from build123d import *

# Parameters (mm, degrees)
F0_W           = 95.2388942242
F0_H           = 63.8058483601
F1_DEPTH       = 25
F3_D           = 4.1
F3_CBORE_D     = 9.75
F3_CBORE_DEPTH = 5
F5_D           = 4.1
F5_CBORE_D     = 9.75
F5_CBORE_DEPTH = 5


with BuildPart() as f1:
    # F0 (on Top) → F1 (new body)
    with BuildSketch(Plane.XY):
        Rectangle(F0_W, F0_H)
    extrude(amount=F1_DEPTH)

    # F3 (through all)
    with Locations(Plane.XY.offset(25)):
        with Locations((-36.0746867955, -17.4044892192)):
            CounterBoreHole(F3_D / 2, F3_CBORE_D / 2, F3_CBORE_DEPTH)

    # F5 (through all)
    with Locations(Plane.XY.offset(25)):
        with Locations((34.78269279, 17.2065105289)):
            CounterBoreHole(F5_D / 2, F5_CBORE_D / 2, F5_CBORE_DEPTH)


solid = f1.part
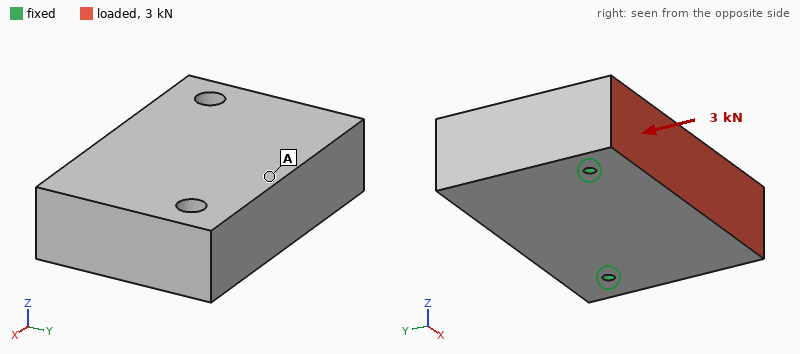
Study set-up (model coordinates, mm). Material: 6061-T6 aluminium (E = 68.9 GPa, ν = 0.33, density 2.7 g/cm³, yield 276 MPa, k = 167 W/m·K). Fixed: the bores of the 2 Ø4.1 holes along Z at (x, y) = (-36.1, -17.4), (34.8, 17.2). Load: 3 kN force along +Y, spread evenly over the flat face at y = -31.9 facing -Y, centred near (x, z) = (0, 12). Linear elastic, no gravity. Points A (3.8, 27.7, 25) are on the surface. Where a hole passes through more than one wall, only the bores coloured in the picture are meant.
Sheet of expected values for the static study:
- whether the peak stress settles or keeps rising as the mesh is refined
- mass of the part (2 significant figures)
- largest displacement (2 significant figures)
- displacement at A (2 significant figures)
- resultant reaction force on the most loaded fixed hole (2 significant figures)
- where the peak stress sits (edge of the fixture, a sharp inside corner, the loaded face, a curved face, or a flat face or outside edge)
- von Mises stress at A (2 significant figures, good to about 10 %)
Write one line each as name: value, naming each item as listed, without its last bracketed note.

whether the peak stress settles or keeps rising as the mesh is refined: keeps rising
mass of the part: 410 g
largest displacement: 2.2 µm
displacement at A: 1.6 µm
resultant reaction force on the most loaded fixed hole: 1.5 kN
where the peak stress sits: edge of the fixture
von Mises stress at A: 0.99 MPa
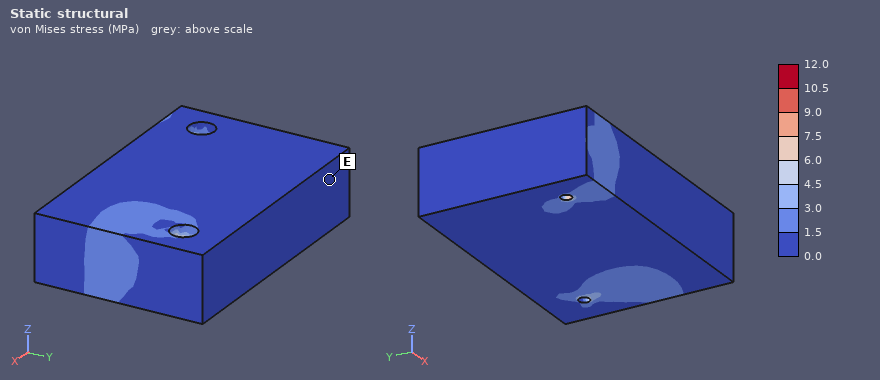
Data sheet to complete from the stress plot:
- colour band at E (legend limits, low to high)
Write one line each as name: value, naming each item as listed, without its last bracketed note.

colour band at E: 0.0 to 1.5 MPa
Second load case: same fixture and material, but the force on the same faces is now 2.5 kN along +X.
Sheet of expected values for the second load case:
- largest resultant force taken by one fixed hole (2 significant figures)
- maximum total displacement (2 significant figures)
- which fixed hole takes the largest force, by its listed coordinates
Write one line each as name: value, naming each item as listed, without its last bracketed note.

largest resultant force taken by one fixed hole: 2.0 kN
maximum total displacement: 3.7 µm
which fixed hole takes the largest force, by its listed coordinates: (-36.1, -17.4)
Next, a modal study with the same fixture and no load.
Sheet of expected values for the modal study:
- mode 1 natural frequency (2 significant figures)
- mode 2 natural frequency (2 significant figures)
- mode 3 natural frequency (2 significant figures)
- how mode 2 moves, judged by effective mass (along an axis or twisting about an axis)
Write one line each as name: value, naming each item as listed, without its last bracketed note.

mode 1 natural frequency: 4900 Hz
mode 2 natural frequency: 7100 Hz
mode 3 natural frequency: 12 kHz
how mode 2 moves, judged by effective mass: along Z
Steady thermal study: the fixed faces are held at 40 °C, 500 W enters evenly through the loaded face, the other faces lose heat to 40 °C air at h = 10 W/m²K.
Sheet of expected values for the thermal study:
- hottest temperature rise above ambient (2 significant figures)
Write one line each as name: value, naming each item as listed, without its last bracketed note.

hottest temperature rise above ambient: 71 K
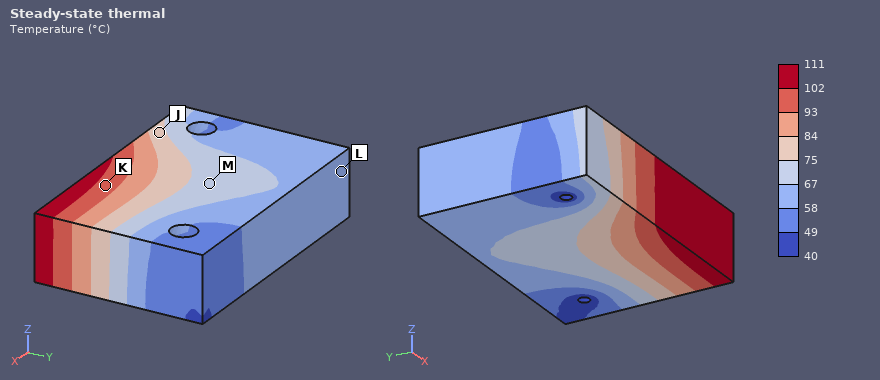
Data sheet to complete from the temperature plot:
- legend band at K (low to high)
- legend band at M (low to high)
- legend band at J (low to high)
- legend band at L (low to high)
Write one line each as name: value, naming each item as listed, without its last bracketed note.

legend band at K: 93 to 102 °C
legend band at M: 67 to 75 °C
legend band at J: 75 to 84 °C
legend band at L: 58 to 67 °C
